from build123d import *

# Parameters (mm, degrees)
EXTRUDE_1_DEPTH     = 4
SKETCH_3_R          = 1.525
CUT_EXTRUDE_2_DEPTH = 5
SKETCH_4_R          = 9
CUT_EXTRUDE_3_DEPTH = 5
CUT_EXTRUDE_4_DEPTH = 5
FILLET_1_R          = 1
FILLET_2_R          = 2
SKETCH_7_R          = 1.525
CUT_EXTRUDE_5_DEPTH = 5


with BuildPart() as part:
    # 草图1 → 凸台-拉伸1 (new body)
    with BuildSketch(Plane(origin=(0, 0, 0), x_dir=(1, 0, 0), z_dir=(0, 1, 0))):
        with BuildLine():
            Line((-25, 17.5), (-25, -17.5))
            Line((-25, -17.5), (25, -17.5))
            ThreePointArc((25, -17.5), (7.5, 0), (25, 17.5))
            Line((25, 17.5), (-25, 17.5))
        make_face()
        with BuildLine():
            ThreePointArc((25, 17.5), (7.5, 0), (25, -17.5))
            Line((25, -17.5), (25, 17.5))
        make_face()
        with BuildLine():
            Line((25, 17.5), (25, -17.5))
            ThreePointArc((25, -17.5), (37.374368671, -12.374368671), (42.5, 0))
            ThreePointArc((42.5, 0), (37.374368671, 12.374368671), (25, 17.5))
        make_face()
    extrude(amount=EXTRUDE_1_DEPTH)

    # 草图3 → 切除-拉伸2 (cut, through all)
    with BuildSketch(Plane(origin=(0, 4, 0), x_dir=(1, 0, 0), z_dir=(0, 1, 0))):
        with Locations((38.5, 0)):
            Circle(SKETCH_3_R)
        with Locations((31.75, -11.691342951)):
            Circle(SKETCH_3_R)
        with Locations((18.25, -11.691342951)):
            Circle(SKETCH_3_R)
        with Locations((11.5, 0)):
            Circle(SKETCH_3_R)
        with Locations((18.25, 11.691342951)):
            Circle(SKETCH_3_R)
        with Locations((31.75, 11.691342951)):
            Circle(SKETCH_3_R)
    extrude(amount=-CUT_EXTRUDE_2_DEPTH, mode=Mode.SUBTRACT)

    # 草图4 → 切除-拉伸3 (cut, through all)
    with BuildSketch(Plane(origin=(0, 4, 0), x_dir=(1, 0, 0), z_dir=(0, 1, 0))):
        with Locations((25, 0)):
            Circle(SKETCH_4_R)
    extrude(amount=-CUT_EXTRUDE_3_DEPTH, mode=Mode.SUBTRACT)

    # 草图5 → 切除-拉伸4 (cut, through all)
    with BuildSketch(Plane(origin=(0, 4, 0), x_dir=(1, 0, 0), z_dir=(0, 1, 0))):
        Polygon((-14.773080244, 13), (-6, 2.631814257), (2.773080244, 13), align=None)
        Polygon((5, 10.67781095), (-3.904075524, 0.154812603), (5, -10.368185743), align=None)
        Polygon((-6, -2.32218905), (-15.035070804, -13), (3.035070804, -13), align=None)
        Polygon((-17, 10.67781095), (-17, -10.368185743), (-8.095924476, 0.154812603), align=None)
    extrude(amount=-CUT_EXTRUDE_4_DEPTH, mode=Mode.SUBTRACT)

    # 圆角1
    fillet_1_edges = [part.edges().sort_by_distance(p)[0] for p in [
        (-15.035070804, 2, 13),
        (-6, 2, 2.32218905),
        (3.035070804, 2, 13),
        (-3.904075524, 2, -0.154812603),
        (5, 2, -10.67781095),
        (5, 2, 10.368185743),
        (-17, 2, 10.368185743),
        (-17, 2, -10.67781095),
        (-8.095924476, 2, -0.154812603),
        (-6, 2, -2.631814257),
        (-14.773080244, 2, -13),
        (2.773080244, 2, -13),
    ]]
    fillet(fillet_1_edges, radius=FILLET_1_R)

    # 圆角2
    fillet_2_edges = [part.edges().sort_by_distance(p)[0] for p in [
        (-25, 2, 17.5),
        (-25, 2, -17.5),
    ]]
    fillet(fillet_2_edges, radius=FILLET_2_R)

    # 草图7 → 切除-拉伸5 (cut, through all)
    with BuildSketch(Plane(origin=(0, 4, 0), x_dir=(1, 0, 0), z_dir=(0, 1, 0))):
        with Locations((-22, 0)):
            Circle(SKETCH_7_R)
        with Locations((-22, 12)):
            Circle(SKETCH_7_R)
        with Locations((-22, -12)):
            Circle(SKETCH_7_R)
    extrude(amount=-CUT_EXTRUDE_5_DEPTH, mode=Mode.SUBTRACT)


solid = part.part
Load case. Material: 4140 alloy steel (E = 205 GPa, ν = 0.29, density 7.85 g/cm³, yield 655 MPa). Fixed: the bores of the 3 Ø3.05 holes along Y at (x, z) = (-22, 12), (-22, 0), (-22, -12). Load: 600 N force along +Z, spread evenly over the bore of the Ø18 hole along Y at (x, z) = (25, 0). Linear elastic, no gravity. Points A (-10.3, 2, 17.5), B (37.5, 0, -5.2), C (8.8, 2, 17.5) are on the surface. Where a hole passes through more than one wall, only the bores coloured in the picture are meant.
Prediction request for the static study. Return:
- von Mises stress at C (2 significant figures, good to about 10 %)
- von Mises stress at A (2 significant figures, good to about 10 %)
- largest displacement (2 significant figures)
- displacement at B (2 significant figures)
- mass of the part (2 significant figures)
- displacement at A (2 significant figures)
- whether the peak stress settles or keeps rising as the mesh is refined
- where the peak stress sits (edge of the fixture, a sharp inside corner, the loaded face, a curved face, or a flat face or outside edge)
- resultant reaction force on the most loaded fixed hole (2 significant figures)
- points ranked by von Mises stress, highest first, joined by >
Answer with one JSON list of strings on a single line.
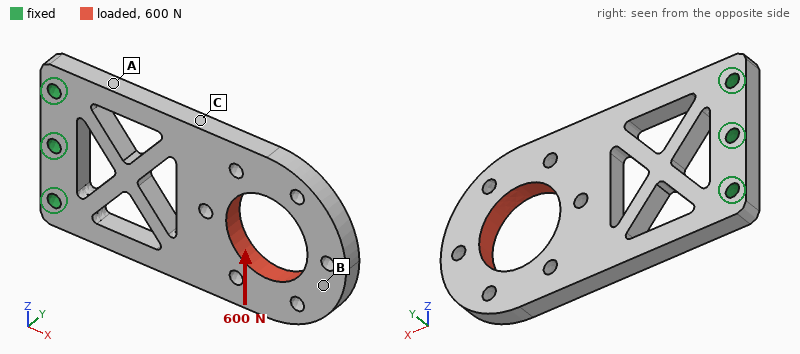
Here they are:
["21 MPa", "38 MPa", "31 µm", "29 µm", "49 g", "6.2 µm", "keeps rising", "edge of the fixture", "1.0 kN", "A > C > B"]
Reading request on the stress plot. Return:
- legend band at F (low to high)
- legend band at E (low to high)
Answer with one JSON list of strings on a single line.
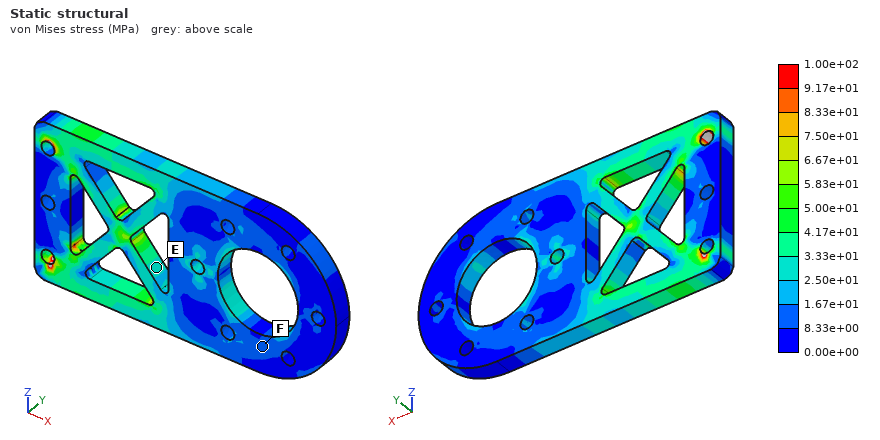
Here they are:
["8.33e+00 to 1.67e+01 MPa", "2.50e+01 to 3.33e+01 MPa"]
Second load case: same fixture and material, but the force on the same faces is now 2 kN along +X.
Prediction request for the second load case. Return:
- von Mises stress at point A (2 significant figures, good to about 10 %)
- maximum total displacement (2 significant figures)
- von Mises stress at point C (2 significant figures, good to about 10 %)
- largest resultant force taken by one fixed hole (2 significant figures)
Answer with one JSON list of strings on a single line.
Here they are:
["28 MPa", "11 µm", "45 MPa", "1.1 kN"]
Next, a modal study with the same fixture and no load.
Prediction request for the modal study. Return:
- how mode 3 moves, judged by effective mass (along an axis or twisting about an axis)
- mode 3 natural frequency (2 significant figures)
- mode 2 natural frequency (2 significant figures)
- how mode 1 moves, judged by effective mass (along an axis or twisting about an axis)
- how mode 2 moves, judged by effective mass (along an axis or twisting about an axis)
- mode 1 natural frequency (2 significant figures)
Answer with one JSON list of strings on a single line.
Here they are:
["along Y", "4400 Hz", "2800 Hz", "along Y", "twisting about X", "700 Hz"]
